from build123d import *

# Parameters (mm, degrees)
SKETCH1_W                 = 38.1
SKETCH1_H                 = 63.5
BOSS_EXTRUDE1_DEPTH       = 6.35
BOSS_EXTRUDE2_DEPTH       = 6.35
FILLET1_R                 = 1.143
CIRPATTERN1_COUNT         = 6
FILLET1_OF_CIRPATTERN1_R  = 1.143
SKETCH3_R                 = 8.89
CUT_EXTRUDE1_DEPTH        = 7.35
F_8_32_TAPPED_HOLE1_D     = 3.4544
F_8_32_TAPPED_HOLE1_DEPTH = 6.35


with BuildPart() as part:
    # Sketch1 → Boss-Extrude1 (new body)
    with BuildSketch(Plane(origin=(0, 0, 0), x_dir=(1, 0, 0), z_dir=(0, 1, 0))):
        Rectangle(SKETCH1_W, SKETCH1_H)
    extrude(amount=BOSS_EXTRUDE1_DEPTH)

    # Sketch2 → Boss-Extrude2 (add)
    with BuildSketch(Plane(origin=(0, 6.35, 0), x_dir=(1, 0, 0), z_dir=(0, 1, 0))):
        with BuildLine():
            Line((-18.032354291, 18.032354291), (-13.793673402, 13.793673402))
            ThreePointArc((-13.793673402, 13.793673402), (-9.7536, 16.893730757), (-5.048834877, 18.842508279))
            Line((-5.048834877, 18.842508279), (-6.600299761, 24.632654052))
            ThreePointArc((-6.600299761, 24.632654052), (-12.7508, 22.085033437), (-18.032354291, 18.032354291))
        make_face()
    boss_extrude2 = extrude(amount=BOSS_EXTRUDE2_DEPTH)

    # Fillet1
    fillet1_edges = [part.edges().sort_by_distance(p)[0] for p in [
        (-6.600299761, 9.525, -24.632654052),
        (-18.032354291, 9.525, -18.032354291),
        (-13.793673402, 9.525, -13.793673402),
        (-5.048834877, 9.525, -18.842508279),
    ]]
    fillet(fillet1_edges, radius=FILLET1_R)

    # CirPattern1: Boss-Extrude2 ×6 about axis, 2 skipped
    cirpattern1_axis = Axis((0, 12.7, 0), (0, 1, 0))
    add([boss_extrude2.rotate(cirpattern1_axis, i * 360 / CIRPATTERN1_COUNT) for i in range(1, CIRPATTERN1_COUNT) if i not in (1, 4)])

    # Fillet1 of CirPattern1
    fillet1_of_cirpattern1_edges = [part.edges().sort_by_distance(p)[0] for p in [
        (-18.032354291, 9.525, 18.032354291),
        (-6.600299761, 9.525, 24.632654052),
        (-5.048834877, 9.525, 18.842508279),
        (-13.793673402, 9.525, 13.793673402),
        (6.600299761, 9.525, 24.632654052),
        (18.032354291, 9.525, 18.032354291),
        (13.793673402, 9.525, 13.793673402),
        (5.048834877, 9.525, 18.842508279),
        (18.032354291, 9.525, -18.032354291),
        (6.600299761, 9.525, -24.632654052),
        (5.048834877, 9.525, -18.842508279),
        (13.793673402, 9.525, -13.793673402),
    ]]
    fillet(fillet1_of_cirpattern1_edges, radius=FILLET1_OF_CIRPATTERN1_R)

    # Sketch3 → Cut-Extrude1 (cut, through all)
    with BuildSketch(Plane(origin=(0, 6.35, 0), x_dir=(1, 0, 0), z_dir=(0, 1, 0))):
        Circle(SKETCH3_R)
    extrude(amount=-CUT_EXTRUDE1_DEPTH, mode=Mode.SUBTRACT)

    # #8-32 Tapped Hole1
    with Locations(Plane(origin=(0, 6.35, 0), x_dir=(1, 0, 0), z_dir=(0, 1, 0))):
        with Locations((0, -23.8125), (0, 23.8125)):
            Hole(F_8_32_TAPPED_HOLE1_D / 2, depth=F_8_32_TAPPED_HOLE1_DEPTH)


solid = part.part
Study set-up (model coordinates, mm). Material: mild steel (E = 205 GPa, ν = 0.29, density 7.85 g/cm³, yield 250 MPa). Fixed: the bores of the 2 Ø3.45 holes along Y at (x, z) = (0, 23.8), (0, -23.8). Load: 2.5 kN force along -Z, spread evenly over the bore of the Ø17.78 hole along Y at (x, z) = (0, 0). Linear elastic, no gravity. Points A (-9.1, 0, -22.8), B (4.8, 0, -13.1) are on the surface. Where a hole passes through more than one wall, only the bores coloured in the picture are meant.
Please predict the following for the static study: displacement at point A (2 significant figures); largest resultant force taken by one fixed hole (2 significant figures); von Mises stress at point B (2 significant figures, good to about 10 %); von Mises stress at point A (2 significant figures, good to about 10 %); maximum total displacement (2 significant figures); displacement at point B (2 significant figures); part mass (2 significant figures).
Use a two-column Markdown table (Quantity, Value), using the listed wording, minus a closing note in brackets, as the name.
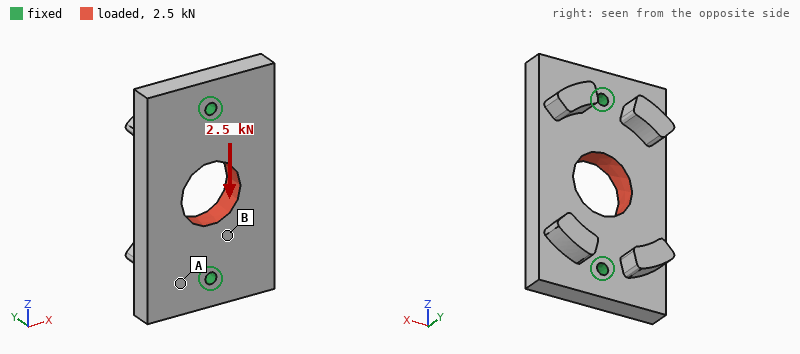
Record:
| Quantity | Value |
|---|---|
| displacement at point A | 0.61 µm |
| largest resultant force taken by one fixed hole | 1.3 kN |
| von Mises stress at point B | 11 MPa |
| von Mises stress at point A | 3.6 MPa |
| maximum total displacement | 1.3 µm |
| displacement at point B | 0.76 µm |
| part mass | 120 g |
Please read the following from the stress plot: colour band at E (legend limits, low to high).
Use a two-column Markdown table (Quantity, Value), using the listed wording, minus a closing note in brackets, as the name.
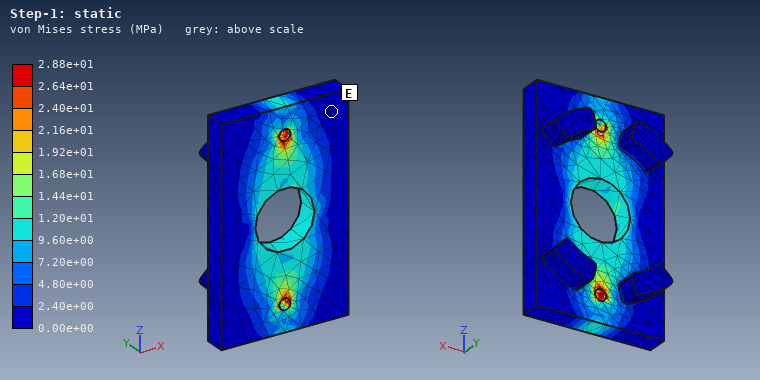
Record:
| Quantity | Value |
|---|---|
| colour band at E | 0.00e+00 to 2.40e+00 MPa |
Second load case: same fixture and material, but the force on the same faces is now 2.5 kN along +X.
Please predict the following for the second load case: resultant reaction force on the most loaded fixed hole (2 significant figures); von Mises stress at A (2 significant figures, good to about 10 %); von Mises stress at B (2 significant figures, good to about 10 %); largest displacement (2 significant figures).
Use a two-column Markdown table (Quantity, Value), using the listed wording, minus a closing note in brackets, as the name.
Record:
| Quantity | Value |
|---|---|
| resultant reaction force on the most loaded fixed hole | 1.3 kN |
| von Mises stress at A | 6.9 MPa |
| von Mises stress at B | 13 MPa |
| largest displacement | 2.7 µm |
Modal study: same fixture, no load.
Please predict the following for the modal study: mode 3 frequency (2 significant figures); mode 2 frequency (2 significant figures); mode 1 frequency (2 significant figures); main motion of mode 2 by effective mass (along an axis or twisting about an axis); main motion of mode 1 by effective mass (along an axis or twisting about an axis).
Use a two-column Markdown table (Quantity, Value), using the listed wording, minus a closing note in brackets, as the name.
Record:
| Quantity | Value |
|---|---|
| mode 3 frequency | 12 kHz |
| mode 2 frequency | 8800 Hz |
| mode 1 frequency | 7200 Hz |
| main motion of mode 2 by effective mass | along Y |
| main motion of mode 1 by effective mass | twisting about Z |
